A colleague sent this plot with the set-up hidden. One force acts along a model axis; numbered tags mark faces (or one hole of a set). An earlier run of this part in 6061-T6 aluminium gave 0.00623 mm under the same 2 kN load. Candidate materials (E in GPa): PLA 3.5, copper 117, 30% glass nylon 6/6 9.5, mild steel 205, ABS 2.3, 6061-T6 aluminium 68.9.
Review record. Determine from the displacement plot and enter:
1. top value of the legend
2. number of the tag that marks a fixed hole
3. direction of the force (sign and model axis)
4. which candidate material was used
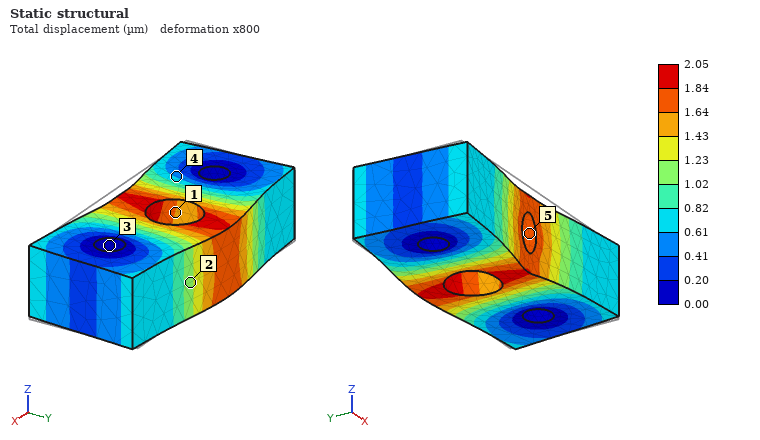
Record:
2.05 µm
3
+Y
mild steel
